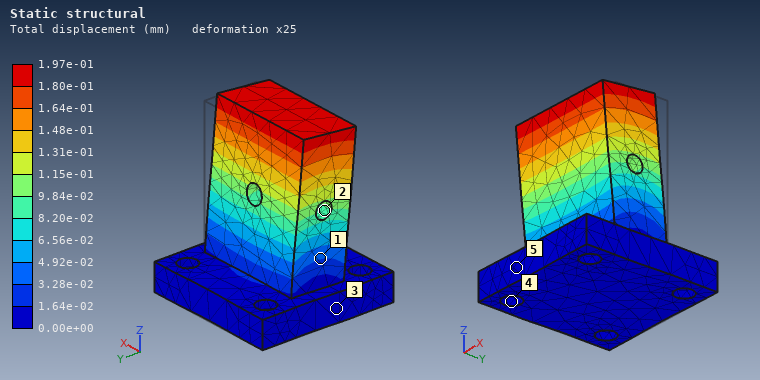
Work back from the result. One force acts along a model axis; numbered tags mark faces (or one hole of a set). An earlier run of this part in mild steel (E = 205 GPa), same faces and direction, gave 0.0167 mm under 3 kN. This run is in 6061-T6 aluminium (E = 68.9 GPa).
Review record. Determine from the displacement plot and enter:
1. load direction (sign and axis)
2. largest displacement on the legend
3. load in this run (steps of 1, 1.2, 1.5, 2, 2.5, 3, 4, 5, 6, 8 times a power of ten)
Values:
-Y
1.97e-01 mm
12 kN
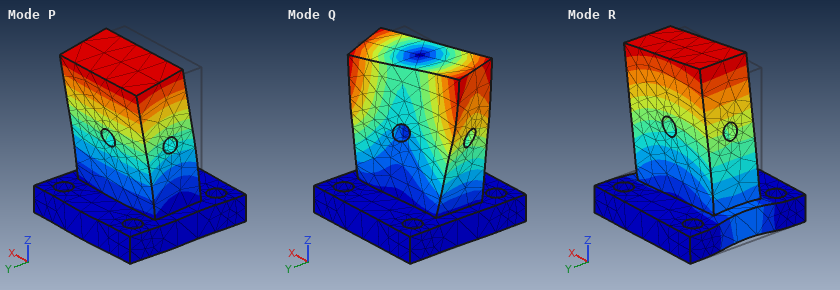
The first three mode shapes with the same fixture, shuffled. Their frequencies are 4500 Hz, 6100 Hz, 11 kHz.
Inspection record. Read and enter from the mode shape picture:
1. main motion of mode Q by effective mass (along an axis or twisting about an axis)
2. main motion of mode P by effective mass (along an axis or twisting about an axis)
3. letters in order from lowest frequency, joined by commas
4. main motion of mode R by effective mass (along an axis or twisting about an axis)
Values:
twisting about Z
along Y
P, R, Q
along X
